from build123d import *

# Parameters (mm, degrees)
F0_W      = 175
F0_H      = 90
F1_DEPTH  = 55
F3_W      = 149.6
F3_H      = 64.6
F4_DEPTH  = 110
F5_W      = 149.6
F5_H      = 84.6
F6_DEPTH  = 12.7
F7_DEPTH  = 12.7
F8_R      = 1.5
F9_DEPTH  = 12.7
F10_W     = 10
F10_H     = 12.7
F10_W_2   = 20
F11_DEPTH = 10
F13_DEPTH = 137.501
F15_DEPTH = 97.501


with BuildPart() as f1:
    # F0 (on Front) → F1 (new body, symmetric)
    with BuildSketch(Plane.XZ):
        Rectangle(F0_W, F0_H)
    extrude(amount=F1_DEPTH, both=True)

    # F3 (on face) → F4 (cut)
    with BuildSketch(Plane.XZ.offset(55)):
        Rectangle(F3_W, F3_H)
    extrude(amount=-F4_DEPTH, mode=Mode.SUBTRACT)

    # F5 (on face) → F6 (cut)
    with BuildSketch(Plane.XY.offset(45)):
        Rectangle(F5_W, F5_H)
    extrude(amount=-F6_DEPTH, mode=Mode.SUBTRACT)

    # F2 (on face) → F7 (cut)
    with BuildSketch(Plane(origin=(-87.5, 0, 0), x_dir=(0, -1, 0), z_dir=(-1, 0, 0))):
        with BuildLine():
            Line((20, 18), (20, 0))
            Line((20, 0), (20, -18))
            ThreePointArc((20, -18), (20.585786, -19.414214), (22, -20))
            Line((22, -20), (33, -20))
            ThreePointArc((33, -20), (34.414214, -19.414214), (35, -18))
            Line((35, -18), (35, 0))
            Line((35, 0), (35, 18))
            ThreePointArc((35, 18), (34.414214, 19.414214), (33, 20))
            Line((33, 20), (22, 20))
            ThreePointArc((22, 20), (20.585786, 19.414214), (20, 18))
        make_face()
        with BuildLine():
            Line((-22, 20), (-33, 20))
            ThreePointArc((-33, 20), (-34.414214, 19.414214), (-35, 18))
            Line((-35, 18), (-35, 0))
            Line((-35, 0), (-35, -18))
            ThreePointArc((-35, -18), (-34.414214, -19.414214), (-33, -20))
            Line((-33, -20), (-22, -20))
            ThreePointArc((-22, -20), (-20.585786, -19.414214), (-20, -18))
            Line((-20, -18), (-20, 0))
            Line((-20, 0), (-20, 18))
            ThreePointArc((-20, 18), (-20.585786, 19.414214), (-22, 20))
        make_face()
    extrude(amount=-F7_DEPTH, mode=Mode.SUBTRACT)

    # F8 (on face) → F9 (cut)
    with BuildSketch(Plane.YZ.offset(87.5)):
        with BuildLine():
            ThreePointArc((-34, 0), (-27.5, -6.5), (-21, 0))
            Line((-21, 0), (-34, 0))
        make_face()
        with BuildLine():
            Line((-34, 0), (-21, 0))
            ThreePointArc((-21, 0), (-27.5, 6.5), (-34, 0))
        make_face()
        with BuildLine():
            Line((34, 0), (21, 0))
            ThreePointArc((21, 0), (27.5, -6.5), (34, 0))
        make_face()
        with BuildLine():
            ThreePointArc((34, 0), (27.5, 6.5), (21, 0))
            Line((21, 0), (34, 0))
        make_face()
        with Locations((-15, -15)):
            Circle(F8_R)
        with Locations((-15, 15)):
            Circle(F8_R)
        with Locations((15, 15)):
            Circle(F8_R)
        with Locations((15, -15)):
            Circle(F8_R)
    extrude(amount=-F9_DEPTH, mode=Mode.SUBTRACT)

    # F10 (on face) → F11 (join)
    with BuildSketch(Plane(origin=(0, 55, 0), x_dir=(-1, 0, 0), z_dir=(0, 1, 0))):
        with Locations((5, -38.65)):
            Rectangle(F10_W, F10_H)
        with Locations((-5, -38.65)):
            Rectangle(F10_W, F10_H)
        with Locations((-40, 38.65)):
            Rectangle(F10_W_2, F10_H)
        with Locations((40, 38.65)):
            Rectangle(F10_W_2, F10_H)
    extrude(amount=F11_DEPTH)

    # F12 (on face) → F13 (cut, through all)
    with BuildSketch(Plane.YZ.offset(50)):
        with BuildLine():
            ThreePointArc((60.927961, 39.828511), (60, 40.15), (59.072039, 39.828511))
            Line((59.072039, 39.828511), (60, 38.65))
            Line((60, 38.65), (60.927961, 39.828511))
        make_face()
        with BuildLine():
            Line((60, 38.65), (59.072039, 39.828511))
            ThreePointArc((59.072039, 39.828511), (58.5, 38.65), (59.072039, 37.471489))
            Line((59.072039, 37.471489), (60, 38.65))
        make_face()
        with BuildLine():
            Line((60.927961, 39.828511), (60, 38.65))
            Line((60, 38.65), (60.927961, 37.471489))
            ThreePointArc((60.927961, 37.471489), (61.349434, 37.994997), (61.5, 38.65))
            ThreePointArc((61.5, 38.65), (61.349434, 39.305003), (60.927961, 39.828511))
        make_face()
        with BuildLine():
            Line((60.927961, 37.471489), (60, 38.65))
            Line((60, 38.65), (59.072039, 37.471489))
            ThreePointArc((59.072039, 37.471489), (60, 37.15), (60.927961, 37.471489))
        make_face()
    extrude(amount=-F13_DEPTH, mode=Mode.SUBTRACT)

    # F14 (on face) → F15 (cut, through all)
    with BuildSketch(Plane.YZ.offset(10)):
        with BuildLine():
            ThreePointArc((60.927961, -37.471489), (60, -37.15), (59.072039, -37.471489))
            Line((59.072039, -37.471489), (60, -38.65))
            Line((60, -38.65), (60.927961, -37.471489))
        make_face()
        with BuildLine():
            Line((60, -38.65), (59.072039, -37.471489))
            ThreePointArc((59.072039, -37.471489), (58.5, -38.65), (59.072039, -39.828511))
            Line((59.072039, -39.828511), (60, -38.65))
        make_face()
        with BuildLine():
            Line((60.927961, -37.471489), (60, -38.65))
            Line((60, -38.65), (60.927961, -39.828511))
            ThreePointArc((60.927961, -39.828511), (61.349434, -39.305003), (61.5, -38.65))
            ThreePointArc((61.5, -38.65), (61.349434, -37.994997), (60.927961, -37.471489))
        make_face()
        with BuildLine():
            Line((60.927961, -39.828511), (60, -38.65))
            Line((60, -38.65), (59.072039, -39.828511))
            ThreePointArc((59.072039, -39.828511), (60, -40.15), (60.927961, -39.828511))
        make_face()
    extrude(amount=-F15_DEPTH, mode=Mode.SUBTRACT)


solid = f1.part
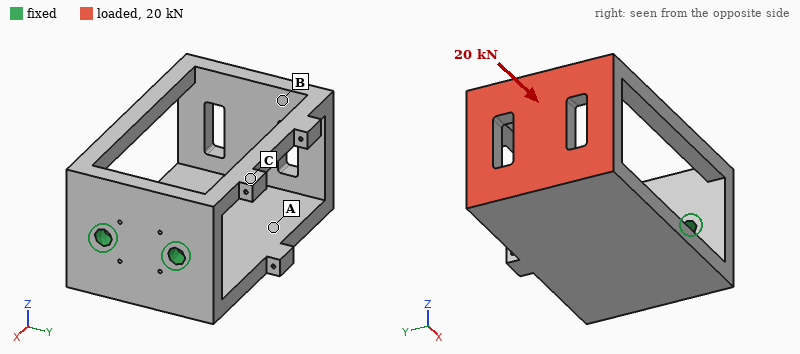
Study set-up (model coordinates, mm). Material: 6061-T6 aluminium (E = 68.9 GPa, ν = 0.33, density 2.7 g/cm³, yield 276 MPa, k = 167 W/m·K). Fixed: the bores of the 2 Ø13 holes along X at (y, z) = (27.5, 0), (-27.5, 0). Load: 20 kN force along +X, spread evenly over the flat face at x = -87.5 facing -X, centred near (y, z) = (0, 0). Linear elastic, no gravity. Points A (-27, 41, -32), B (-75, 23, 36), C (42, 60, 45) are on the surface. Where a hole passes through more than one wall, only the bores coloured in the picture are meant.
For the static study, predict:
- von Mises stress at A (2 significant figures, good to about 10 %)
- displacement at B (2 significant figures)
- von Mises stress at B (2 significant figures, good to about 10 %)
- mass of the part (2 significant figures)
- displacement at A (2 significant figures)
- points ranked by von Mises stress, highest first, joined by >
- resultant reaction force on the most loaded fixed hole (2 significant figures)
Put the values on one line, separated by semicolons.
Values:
29 MPa; 0.38 mm; 64 MPa; 1.3 kg; 0.12 mm; B > A > C; 10 kN
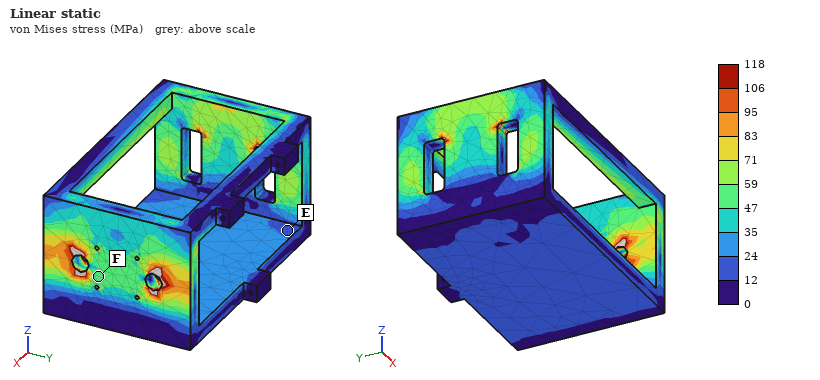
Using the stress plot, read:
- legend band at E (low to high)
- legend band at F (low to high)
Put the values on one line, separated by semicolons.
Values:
12 to 24 MPa; 47 to 59 MPa
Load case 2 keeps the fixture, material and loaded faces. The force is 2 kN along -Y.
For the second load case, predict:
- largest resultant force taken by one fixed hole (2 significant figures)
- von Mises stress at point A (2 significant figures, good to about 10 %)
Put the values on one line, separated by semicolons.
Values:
4.6 kN; 13 MPa
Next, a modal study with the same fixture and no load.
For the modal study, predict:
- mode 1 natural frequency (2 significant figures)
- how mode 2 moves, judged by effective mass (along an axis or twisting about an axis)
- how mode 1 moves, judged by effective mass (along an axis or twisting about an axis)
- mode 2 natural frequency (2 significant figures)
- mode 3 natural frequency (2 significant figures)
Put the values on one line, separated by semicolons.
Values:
290 Hz; along Y; along Z; 450 Hz; 850 Hz
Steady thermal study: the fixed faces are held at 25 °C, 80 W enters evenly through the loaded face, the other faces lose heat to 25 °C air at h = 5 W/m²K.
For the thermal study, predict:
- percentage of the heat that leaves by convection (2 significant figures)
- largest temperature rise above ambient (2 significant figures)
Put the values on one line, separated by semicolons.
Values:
14 %; 55 K
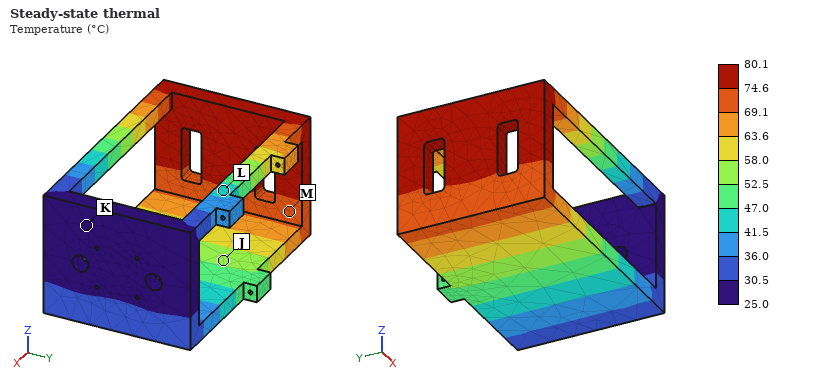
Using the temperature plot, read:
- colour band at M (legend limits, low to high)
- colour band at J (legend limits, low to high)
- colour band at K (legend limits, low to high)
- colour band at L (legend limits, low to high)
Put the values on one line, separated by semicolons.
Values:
69.1 to 74.6 °C; 52.5 to 58.0 °C; 25.0 to 30.5 °C; 41.5 to 47.0 °C
